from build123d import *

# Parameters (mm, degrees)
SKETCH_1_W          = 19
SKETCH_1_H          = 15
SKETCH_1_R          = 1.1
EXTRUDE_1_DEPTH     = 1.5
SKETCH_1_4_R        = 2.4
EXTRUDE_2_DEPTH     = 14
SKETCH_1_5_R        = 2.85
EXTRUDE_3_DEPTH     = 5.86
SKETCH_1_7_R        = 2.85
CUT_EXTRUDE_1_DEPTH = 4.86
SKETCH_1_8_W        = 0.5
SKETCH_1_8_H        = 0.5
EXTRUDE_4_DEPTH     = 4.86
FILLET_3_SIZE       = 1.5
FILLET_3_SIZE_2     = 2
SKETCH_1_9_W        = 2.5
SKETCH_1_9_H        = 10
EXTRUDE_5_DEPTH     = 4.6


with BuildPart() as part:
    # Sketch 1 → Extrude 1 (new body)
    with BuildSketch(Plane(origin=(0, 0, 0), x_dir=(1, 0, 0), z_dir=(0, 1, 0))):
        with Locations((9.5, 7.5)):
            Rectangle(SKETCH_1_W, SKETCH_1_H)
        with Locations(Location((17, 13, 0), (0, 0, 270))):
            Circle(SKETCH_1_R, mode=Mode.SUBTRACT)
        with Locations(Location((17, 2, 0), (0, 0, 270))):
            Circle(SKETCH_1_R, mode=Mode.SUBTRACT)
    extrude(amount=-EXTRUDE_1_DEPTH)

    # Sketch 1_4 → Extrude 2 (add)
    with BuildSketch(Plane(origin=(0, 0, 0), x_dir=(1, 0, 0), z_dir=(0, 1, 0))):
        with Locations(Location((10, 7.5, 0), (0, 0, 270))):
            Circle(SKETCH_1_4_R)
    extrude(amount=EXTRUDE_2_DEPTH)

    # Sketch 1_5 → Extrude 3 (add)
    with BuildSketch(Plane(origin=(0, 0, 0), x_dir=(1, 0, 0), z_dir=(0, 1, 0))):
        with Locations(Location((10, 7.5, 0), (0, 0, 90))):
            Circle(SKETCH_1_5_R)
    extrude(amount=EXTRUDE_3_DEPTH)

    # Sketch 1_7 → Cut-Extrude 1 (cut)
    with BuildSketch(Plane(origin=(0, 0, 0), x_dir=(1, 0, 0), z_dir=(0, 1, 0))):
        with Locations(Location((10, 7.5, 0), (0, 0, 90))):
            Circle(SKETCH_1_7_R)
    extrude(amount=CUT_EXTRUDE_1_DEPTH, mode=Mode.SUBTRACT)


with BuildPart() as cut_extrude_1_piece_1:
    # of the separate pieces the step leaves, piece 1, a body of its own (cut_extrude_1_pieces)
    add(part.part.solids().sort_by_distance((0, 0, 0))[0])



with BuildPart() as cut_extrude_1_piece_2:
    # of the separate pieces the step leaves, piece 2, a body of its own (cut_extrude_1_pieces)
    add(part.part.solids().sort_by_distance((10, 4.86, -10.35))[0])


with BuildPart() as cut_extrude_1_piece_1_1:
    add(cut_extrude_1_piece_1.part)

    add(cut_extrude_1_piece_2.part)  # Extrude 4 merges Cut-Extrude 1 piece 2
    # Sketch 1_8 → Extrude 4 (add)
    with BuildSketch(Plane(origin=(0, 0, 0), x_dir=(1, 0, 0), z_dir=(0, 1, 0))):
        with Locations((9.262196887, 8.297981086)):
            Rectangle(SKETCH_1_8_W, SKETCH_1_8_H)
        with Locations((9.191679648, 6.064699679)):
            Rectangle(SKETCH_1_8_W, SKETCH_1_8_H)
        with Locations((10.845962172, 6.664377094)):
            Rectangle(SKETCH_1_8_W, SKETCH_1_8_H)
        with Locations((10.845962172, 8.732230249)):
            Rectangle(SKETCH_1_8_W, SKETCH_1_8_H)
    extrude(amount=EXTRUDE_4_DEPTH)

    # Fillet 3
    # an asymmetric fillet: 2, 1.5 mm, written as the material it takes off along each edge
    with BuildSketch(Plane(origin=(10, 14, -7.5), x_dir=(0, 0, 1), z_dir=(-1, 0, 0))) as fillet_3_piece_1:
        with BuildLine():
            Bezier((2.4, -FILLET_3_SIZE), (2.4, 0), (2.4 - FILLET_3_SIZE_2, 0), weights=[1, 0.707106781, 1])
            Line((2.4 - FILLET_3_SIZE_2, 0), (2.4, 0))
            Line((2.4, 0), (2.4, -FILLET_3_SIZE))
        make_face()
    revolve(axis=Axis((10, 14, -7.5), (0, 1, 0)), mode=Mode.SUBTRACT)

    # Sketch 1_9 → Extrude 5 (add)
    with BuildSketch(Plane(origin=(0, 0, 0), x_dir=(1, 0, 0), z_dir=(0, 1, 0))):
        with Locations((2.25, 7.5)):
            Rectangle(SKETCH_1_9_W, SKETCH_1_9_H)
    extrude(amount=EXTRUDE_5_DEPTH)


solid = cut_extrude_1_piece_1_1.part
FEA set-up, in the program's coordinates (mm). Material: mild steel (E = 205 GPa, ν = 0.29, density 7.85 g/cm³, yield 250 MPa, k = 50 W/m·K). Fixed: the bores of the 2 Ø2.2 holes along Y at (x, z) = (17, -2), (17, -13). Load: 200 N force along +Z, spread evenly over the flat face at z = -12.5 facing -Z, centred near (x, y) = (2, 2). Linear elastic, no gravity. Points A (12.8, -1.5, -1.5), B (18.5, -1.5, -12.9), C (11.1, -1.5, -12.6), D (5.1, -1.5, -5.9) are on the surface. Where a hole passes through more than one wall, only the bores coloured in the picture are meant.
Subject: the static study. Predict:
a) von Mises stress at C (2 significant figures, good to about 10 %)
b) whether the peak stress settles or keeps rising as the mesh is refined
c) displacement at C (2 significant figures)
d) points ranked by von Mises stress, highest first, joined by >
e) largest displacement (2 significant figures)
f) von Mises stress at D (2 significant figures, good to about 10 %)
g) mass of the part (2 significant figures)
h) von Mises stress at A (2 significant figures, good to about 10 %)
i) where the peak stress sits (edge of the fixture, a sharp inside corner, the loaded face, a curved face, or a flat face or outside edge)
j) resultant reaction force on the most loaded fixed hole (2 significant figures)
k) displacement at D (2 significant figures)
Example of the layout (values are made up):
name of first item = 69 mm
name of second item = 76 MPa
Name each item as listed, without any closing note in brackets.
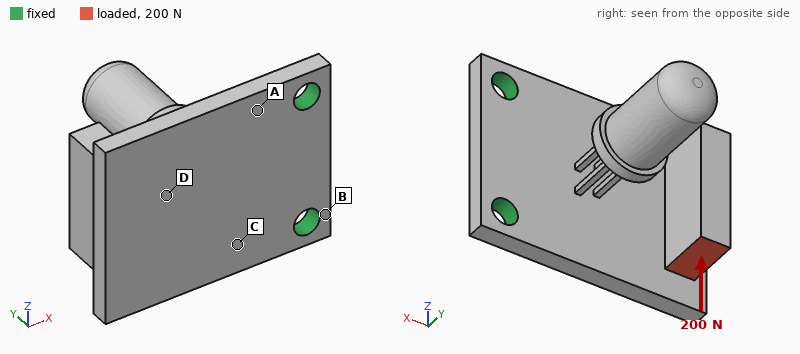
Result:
von Mises stress at C = 67 MPa
whether the peak stress settles or keeps rising as the mesh is refined = keeps rising
displacement at C = 6.2 µm
points ranked by von Mises stress, highest first, joined by > = A > C > D > B
largest displacement = 32 µm
von Mises stress at D = 43 MPa
mass of the part = 5.5 g
von Mises stress at A = 84 MPa
where the peak stress sits = edge of the fixture
resultant reaction force on the most loaded fixed hole = 270 N
displacement at D = 5.7 µm
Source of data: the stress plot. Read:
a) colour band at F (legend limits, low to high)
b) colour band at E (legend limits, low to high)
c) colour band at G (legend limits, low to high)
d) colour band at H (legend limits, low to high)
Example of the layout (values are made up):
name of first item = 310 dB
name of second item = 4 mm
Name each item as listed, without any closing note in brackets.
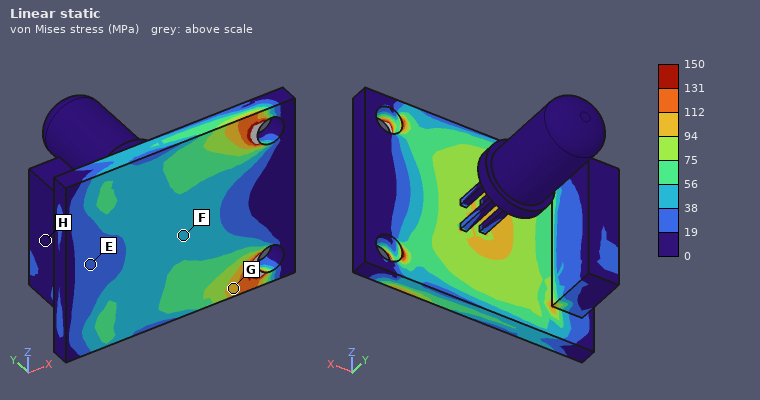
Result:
colour band at F = 38 to 56 MPa
colour band at E = 19 to 38 MPa
colour band at G = 94 to 112 MPa
colour band at H = 0 to 19 MPa
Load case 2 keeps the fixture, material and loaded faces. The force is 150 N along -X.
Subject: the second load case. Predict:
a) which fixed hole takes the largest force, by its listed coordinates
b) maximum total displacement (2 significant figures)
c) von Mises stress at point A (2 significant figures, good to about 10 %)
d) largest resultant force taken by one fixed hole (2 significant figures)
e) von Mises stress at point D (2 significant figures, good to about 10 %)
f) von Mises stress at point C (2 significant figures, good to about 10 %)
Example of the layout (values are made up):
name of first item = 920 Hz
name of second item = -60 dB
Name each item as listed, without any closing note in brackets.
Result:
which fixed hole takes the largest force, by its listed coordinates = (17, -13)
maximum total displacement = 79 µm
von Mises stress at point A = 86 MPa
largest resultant force taken by one fixed hole = 140 N
von Mises stress at point D = 72 MPa
von Mises stress at point C = 64 MPa
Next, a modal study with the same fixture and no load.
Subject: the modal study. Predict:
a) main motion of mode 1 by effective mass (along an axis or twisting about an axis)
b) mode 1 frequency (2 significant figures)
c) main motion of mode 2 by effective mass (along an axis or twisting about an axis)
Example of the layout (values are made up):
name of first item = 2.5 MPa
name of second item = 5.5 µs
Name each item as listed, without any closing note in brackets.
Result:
main motion of mode 1 by effective mass = along X
mode 1 frequency = 1800 Hz
main motion of mode 2 by effective mass = along Z
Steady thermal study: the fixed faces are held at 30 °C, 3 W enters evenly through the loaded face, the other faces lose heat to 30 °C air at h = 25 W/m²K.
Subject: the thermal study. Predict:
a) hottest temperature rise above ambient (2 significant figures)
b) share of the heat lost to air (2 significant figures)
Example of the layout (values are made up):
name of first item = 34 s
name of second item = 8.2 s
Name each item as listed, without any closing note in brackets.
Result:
hottest temperature rise above ambient = 55 K
share of the heat lost to air = 15 %
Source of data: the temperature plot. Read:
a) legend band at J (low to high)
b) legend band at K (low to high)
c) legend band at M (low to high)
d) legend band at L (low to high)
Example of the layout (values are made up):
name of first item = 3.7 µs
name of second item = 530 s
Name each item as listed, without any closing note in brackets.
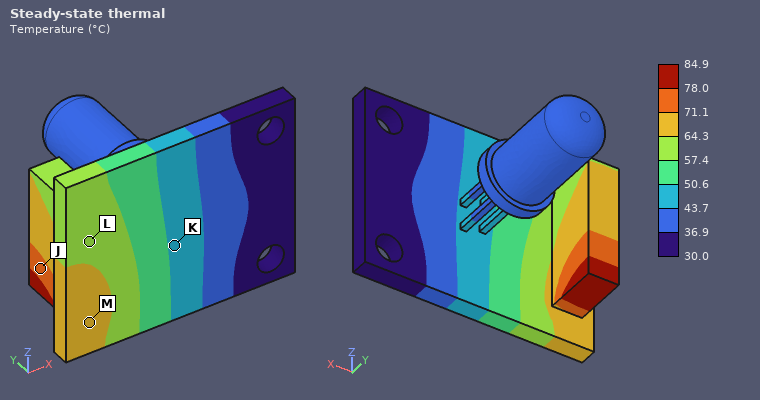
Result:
legend band at J = 71.1 to 78.0 °C
legend band at K = 43.7 to 50.6 °C
legend band at M = 64.3 to 71.1 °C
legend band at L = 57.4 to 64.3 °C
